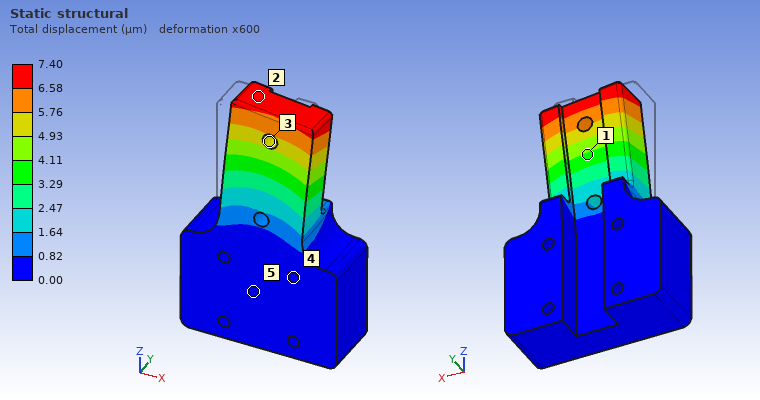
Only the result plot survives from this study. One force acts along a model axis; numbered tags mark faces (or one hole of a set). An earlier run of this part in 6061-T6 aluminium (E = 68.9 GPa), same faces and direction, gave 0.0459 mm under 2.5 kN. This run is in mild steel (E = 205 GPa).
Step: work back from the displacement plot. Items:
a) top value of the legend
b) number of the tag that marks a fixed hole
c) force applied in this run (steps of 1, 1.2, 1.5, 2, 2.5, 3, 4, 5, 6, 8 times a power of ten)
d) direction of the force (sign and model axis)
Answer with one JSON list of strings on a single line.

["7.40 µm", "4", "1.2 kN", "+X"]
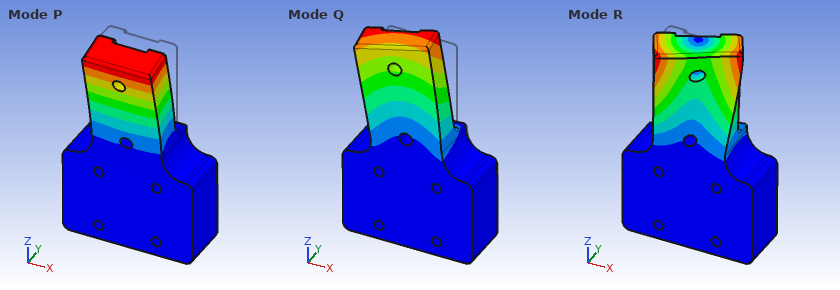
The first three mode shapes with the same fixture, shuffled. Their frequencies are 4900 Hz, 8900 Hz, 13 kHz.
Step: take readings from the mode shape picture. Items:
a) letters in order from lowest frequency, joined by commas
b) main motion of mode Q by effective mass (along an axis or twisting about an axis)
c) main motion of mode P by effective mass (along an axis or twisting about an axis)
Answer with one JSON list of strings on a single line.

["P, Q, R", "along X", "along Y"]
